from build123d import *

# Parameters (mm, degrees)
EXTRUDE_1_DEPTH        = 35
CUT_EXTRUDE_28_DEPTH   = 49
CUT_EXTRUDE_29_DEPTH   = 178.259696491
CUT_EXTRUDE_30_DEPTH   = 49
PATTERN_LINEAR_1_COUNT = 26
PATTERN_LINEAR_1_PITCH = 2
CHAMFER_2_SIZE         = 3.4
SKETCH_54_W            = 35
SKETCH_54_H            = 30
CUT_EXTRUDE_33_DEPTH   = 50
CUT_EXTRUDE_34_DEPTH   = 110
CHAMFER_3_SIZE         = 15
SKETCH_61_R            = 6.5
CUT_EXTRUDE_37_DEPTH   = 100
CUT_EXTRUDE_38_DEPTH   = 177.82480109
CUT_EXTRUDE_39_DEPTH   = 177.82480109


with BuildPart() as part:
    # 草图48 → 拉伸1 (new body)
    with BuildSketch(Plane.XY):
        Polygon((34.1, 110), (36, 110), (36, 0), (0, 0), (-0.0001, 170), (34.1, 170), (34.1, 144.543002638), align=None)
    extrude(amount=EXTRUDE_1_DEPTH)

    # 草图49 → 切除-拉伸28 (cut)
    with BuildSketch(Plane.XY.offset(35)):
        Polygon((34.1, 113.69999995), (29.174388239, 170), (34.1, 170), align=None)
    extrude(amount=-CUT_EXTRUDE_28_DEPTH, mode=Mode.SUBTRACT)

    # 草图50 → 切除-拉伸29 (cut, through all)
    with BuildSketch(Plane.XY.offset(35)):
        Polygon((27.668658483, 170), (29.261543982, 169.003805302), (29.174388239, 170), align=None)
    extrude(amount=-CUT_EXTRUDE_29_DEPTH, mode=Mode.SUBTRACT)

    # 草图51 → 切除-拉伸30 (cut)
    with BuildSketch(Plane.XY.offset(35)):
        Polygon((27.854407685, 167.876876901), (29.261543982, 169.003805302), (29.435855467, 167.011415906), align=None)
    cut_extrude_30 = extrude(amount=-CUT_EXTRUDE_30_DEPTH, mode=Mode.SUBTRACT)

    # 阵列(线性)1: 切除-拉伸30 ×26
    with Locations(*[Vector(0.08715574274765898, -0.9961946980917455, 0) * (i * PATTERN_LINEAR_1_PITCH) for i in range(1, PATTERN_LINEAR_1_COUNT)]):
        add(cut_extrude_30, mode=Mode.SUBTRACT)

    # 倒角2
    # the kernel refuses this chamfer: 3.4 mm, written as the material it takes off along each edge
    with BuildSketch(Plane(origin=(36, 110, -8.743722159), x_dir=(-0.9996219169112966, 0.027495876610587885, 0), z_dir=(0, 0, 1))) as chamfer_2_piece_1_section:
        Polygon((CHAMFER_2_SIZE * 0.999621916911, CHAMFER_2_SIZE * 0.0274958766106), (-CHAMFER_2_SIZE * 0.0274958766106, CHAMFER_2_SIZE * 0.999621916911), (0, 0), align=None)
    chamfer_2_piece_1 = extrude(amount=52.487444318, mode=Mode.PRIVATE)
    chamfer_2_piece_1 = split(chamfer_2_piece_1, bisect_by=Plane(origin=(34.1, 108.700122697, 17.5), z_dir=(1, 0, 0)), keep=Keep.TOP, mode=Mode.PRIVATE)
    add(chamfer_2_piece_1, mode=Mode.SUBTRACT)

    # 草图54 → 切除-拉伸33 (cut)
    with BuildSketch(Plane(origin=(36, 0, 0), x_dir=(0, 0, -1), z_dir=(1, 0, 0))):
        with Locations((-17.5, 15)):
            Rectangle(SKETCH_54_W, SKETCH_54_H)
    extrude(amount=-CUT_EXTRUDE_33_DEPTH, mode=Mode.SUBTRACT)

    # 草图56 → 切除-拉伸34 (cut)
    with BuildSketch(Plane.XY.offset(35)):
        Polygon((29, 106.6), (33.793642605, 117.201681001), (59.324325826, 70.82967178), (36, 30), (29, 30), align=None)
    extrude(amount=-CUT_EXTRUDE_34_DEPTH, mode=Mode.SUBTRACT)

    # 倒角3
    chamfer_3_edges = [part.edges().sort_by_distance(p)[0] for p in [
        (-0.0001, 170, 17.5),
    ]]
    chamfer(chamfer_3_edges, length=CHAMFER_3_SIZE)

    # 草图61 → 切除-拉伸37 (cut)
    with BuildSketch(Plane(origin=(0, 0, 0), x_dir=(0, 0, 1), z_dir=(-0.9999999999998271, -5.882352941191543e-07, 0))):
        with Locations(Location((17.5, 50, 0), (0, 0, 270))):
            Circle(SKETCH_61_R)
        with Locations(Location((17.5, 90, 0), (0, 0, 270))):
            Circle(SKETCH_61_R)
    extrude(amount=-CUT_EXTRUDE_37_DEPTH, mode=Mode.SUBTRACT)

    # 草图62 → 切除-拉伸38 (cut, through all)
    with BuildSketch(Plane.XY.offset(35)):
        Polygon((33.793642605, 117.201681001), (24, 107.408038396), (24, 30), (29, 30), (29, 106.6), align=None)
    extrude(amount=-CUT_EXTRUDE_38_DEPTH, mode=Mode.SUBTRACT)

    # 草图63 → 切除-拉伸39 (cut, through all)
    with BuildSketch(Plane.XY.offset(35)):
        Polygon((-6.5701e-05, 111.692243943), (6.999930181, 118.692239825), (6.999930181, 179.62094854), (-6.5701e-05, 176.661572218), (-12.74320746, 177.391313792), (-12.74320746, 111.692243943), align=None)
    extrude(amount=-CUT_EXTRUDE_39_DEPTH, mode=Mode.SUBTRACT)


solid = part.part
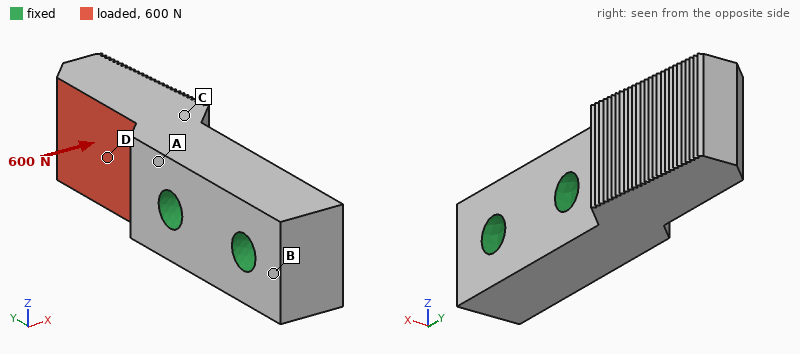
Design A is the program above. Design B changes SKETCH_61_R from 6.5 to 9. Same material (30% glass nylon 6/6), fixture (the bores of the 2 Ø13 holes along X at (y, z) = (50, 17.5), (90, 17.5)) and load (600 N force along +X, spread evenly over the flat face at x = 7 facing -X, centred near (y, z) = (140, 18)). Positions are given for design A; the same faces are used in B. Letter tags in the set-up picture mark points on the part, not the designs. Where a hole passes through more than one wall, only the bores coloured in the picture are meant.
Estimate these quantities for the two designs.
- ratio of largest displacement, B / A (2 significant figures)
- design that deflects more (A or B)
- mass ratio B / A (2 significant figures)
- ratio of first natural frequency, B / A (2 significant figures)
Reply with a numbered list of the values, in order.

1. 0.86
2. A
3. 0.95
4. 1.1
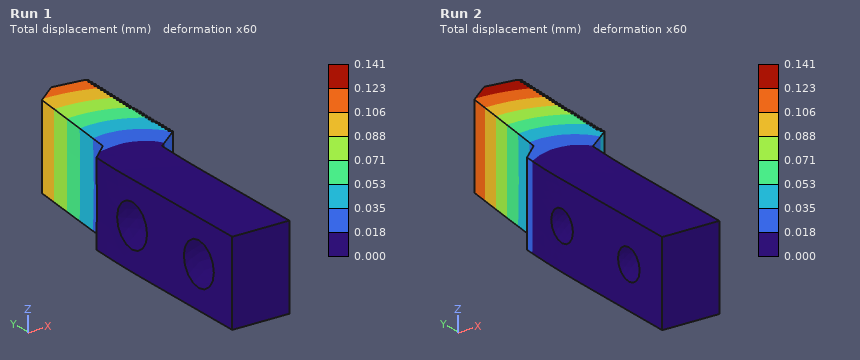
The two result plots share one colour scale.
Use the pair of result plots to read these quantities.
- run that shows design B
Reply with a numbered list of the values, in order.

1. Run 1
